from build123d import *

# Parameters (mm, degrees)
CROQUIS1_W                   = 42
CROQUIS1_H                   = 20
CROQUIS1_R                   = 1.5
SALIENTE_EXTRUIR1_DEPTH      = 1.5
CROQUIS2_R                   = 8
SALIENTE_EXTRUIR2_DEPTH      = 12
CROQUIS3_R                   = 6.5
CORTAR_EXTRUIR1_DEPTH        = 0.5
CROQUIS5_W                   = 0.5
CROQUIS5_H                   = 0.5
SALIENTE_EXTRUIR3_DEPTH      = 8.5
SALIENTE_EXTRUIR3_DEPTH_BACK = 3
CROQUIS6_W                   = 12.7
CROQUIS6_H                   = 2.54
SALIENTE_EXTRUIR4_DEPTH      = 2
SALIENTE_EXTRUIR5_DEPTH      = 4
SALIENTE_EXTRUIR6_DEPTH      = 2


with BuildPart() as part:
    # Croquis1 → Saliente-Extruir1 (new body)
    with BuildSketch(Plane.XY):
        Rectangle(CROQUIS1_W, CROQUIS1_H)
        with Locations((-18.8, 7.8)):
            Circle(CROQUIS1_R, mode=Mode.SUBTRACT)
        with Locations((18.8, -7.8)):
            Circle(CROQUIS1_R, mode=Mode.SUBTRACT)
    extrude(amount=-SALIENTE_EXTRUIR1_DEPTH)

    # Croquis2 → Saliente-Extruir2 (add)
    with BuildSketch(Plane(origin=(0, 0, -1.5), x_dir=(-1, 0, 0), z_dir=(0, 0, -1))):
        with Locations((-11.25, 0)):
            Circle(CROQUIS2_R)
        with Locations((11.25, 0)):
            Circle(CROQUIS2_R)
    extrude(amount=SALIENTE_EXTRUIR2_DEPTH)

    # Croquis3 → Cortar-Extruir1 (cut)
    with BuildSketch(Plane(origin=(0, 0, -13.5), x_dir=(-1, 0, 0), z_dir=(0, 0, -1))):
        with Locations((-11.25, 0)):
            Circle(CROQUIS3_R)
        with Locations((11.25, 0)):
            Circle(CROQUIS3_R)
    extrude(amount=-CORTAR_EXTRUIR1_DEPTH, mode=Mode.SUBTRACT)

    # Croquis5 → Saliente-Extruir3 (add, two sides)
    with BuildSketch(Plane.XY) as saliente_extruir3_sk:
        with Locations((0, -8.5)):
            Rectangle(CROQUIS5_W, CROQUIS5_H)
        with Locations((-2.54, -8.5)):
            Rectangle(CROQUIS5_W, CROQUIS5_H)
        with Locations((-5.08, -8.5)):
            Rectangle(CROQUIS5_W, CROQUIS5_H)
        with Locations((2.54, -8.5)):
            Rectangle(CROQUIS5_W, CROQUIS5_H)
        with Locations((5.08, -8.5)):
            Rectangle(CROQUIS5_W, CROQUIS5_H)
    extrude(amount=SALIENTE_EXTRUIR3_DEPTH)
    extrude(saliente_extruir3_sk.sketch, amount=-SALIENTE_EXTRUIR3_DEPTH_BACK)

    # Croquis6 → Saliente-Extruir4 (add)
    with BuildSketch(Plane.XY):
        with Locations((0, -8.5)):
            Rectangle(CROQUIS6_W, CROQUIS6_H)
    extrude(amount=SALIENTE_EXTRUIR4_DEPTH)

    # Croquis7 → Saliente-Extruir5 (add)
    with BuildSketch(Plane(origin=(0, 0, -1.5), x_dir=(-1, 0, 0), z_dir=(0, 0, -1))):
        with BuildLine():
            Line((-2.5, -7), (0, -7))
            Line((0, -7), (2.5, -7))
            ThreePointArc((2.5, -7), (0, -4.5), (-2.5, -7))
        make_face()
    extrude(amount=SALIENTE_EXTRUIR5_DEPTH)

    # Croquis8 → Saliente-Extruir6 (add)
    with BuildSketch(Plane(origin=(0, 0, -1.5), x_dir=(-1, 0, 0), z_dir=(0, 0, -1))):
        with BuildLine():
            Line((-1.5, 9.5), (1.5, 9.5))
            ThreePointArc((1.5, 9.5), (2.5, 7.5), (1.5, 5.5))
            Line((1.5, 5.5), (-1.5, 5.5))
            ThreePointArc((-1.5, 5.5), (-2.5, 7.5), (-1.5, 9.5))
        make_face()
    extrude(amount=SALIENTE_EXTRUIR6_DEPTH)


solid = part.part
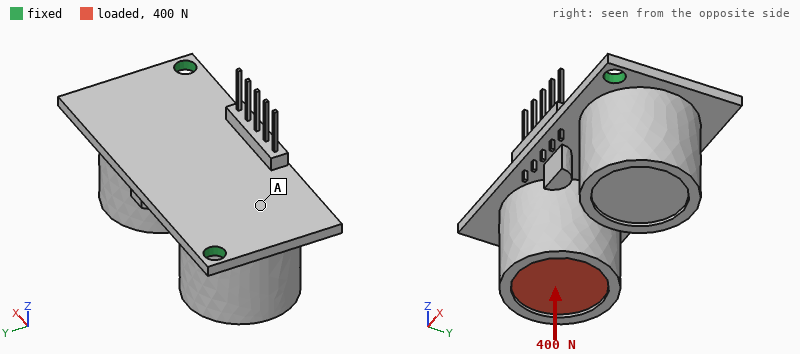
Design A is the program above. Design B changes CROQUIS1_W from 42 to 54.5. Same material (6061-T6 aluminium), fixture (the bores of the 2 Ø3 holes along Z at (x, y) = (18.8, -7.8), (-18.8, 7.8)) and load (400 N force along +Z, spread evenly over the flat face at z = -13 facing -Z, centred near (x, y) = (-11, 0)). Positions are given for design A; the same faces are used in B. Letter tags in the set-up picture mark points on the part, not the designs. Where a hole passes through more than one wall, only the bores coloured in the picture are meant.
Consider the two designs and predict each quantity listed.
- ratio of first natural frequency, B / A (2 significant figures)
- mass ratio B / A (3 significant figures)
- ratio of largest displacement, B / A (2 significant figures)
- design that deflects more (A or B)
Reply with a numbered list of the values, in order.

1. 1.0
2. 1.06
3. 0.91
4. A
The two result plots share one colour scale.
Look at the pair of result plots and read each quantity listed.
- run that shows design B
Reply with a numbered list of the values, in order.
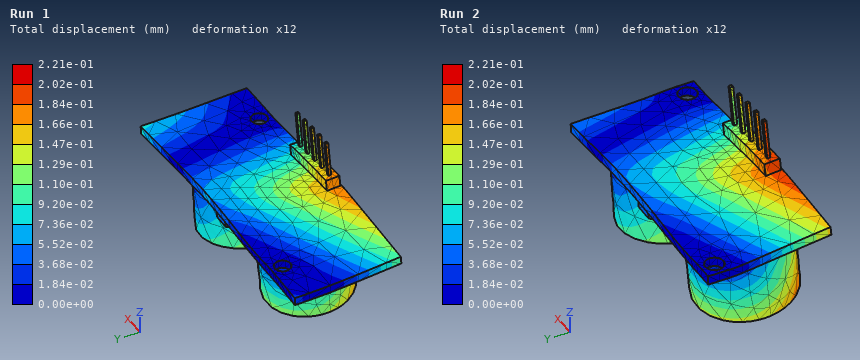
1. Run 1
